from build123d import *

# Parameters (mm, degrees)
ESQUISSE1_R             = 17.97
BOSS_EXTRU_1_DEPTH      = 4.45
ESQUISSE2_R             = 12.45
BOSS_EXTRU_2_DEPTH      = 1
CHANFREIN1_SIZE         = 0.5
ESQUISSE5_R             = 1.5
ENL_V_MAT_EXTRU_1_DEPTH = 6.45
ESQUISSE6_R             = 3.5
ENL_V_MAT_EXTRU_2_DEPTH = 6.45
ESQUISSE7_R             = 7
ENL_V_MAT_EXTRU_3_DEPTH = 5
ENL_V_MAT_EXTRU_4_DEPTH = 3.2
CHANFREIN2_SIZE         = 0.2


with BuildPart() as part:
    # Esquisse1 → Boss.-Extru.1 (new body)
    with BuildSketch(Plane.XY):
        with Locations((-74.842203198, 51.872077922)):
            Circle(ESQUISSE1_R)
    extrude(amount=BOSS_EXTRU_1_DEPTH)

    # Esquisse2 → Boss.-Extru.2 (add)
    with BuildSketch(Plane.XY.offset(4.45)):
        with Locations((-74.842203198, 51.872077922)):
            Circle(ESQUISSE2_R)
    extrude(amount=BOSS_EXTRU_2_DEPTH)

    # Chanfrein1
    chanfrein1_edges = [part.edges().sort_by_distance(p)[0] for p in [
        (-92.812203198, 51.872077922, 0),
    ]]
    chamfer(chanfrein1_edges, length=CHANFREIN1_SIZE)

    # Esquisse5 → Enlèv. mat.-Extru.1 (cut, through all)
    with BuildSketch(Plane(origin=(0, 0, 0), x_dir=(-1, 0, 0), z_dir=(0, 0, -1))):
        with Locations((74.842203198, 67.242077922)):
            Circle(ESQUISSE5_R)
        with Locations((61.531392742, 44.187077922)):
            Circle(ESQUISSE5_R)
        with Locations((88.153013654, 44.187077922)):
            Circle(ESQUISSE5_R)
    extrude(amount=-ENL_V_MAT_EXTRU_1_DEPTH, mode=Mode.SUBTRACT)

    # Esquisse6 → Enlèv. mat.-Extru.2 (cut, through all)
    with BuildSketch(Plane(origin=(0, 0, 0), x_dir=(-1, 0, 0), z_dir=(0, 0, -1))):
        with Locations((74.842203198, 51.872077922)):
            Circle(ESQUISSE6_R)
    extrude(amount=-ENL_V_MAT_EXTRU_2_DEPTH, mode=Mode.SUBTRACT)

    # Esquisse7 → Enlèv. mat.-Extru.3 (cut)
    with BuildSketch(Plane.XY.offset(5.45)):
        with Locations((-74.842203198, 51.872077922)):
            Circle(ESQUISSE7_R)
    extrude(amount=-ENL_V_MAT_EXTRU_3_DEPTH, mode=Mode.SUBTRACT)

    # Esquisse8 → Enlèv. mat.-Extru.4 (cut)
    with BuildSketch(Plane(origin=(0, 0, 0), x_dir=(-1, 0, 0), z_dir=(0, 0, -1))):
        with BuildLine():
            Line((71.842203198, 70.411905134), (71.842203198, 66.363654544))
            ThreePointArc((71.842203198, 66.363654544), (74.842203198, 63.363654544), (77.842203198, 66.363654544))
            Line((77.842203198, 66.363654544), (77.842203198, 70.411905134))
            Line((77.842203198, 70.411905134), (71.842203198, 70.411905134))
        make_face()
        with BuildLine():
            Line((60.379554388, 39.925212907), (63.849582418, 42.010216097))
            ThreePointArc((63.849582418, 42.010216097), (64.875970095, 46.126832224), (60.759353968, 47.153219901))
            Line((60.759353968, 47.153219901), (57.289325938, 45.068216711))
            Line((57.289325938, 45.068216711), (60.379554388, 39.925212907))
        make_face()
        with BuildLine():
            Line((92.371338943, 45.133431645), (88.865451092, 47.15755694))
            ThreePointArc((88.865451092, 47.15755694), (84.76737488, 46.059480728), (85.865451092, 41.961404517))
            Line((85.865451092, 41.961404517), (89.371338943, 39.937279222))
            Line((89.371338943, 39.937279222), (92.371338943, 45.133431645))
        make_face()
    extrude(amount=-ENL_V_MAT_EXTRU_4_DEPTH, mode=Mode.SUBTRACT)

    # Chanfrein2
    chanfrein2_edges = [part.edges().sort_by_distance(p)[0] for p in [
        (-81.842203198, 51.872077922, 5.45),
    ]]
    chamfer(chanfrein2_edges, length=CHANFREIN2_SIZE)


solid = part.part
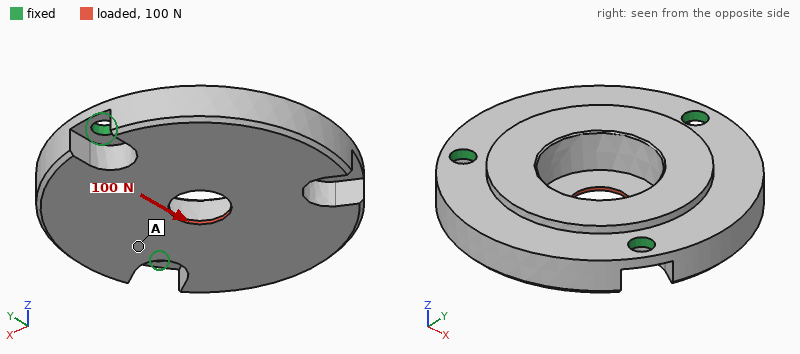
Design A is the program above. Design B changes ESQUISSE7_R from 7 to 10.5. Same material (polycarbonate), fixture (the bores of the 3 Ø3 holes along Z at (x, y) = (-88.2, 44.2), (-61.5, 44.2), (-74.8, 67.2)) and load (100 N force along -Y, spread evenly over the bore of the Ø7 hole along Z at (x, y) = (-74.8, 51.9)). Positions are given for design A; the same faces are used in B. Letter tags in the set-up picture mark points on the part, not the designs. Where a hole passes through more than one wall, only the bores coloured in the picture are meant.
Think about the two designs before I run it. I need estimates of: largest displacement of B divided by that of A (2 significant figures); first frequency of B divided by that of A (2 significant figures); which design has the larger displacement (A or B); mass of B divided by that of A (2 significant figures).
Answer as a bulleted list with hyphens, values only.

- 1.8
- 0.92
- B
- 0.75
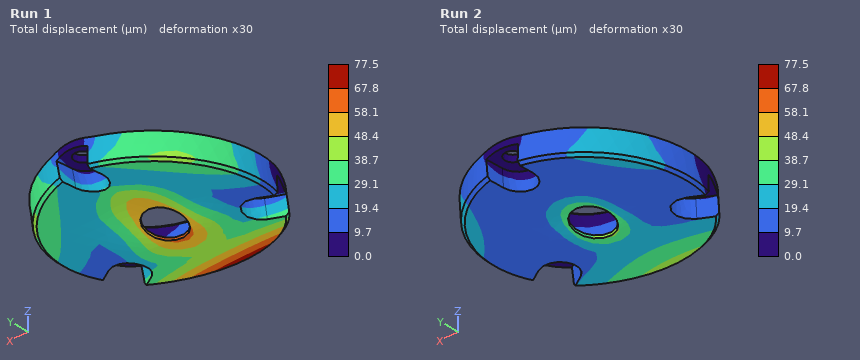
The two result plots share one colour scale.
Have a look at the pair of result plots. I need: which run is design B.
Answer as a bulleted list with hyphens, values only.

- Run 1
